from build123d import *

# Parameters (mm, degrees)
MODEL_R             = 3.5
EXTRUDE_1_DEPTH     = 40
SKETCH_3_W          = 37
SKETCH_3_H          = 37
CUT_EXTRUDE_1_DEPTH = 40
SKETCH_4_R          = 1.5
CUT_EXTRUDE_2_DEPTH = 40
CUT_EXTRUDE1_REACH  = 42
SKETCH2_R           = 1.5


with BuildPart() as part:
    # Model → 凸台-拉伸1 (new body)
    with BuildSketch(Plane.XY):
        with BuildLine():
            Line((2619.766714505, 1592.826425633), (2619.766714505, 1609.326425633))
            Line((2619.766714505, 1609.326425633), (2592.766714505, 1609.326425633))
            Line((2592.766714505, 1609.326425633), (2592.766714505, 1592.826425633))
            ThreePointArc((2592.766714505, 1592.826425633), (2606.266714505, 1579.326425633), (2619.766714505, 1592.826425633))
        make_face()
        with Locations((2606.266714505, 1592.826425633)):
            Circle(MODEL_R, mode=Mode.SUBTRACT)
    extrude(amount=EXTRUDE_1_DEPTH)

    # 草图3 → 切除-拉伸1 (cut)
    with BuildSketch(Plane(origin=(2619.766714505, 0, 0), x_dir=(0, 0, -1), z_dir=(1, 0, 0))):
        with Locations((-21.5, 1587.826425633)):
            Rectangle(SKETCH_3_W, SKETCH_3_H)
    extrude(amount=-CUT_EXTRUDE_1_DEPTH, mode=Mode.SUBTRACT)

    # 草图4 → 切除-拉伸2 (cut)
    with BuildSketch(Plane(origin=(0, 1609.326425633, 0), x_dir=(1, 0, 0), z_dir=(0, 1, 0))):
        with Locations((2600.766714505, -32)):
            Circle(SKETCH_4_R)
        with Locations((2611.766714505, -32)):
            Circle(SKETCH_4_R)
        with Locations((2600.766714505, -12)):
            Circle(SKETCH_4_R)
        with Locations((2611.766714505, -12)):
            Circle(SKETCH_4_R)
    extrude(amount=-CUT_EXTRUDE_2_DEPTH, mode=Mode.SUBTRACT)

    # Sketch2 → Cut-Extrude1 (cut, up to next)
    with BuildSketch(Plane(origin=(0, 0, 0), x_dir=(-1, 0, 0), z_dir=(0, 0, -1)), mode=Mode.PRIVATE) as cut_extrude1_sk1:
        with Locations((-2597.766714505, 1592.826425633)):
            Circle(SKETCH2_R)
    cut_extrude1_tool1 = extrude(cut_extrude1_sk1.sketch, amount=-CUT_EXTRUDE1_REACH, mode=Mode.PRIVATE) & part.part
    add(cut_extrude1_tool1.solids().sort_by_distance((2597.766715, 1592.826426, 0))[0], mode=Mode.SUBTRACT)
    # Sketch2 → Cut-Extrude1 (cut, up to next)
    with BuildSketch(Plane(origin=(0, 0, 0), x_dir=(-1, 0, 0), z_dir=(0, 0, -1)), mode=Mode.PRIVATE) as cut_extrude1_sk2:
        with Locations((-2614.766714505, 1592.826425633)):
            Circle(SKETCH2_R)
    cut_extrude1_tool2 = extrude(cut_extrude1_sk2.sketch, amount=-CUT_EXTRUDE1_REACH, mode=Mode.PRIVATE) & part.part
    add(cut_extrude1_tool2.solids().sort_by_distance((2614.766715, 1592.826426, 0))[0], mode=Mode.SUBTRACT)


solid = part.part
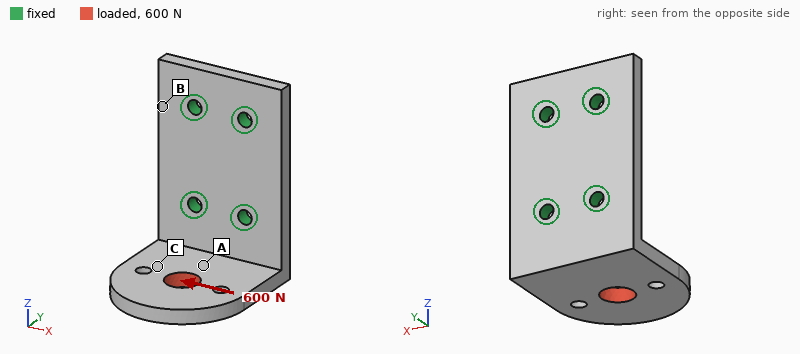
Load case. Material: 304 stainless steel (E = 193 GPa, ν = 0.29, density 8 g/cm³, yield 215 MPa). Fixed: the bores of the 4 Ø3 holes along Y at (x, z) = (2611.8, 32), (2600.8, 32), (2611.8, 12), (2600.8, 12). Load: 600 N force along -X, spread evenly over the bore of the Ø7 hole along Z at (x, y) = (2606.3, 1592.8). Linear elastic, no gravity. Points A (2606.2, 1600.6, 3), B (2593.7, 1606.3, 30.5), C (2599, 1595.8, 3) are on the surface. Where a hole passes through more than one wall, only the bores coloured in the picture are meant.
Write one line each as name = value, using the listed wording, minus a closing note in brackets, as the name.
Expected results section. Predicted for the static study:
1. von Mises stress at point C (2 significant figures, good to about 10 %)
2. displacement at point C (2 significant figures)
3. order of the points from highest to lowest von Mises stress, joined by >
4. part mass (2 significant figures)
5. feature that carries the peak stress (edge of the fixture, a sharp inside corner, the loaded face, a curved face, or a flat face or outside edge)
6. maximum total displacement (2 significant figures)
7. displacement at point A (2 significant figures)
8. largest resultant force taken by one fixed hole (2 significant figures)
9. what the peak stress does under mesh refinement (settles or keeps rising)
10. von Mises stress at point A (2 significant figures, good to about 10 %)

von Mises stress at point C = 35 MPa
displacement at point C = 35 µm
order of the points from highest to lowest von Mises stress, joined by > = A > C > B
part mass = 40 g
feature that carries the peak stress = edge of the fixture
maximum total displacement = 68 µm
displacement at point A = 19 µm
largest resultant force taken by one fixed hole = 750 N
what the peak stress does under mesh refinement = keeps rising
von Mises stress at point A = 50 MPa
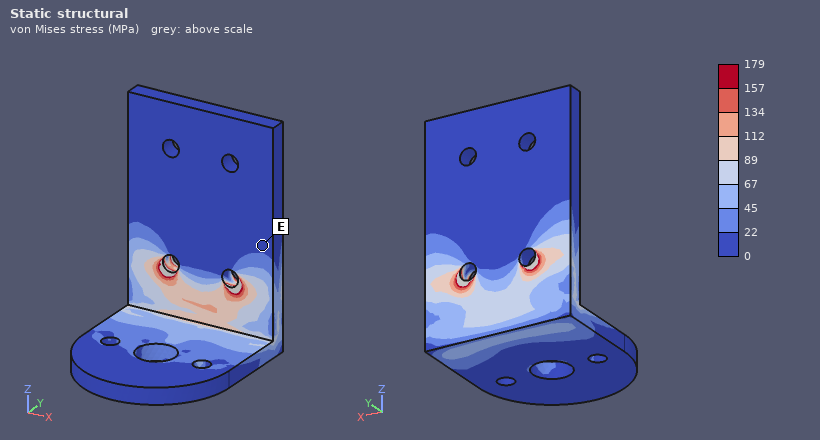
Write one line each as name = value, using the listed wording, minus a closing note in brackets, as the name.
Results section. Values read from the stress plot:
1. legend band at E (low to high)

legend band at E = 0 to 22 MPa
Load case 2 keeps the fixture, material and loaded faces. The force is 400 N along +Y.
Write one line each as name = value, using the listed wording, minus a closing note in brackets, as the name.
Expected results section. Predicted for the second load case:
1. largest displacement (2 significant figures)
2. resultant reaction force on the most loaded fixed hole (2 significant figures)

largest displacement = 54 µm
resultant reaction force on the most loaded fixed hole = 220 N
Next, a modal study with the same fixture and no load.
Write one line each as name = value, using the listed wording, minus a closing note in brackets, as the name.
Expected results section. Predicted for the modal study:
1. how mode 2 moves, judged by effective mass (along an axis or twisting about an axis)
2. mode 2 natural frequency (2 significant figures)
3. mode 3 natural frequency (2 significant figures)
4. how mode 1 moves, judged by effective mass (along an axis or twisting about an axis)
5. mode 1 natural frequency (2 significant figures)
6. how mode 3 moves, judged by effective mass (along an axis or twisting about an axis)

how mode 2 moves, judged by effective mass = along X
mode 2 natural frequency = 4600 Hz
mode 3 natural frequency = 8600 Hz
how mode 1 moves, judged by effective mass = along Z
mode 1 natural frequency = 2300 Hz
how mode 3 moves, judged by effective mass = along Y
